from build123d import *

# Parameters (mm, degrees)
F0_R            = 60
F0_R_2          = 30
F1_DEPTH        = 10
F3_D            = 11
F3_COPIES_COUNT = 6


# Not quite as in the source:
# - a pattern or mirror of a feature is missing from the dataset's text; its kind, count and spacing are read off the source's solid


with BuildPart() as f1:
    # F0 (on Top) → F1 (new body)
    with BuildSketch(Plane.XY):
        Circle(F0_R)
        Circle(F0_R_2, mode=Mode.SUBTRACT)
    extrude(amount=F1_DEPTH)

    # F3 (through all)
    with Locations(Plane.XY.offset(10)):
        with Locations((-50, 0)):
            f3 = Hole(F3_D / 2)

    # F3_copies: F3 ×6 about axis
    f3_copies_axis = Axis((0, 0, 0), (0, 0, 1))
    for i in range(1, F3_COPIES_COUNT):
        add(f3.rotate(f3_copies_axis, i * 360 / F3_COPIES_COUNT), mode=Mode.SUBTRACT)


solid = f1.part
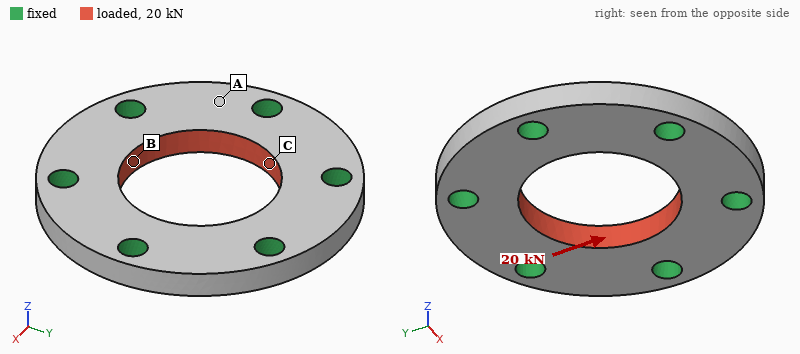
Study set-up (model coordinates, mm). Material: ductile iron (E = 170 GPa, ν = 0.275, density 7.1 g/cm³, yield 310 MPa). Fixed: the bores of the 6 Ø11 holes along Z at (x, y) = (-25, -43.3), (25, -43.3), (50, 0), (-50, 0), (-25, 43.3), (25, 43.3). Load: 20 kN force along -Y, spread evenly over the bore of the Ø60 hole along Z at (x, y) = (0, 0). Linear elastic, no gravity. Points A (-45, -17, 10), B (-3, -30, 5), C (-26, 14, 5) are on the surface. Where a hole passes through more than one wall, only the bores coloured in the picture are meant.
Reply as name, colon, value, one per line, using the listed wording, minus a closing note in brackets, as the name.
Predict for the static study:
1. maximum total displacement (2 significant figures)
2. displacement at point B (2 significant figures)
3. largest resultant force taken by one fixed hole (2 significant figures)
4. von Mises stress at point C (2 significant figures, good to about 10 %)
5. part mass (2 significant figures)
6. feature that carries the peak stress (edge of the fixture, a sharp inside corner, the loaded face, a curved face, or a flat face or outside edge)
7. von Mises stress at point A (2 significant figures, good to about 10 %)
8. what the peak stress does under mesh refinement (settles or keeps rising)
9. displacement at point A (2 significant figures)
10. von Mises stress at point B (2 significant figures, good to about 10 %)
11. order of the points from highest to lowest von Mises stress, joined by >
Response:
maximum total displacement: 2.4 µm
displacement at point B: 2.3 µm
largest resultant force taken by one fixed hole: 3.9 kN
von Mises stress at point C: 17 MPa
part mass: 560 g
feature that carries the peak stress: edge of the fixture
von Mises stress at point A: 4.1 MPa
what the peak stress does under mesh refinement: keeps rising
displacement at point A: 0.71 µm
von Mises stress at point B: 11 MPa
order of the points from highest to lowest von Mises stress, joined by >: C > B > A
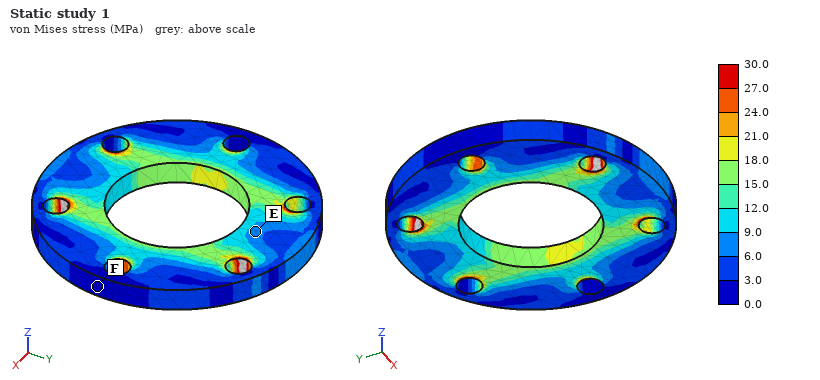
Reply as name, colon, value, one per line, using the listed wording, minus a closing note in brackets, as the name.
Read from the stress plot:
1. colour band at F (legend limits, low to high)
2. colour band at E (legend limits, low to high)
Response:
colour band at F: 0.0 to 3.0 MPa
colour band at E: 6.0 to 9.0 MPa
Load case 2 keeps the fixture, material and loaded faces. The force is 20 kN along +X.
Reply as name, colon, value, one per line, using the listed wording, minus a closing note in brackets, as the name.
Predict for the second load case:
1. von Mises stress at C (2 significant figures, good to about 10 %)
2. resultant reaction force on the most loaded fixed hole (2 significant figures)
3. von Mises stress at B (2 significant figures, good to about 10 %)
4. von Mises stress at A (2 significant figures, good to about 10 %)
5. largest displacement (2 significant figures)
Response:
von Mises stress at C: 13 MPa
resultant reaction force on the most loaded fixed hole: 4.3 kN
von Mises stress at B: 18 MPa
von Mises stress at A: 6.0 MPa
largest displacement: 2.3 µm
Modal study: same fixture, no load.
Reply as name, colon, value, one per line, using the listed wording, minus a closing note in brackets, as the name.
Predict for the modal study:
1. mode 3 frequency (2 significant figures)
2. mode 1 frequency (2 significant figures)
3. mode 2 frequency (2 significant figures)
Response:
mode 3 frequency: 18 kHz
mode 1 frequency: 18 kHz
mode 2 frequency: 18 kHz
